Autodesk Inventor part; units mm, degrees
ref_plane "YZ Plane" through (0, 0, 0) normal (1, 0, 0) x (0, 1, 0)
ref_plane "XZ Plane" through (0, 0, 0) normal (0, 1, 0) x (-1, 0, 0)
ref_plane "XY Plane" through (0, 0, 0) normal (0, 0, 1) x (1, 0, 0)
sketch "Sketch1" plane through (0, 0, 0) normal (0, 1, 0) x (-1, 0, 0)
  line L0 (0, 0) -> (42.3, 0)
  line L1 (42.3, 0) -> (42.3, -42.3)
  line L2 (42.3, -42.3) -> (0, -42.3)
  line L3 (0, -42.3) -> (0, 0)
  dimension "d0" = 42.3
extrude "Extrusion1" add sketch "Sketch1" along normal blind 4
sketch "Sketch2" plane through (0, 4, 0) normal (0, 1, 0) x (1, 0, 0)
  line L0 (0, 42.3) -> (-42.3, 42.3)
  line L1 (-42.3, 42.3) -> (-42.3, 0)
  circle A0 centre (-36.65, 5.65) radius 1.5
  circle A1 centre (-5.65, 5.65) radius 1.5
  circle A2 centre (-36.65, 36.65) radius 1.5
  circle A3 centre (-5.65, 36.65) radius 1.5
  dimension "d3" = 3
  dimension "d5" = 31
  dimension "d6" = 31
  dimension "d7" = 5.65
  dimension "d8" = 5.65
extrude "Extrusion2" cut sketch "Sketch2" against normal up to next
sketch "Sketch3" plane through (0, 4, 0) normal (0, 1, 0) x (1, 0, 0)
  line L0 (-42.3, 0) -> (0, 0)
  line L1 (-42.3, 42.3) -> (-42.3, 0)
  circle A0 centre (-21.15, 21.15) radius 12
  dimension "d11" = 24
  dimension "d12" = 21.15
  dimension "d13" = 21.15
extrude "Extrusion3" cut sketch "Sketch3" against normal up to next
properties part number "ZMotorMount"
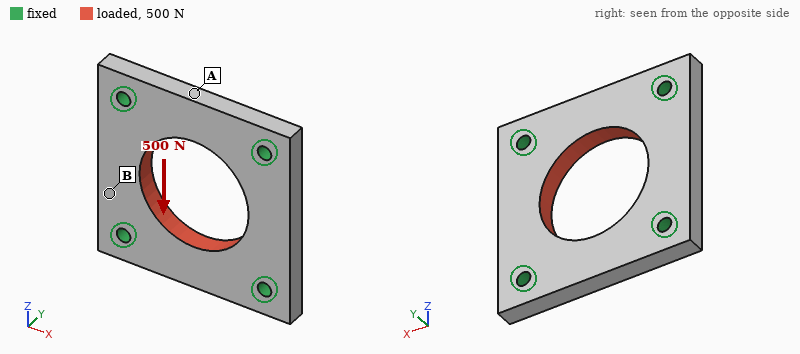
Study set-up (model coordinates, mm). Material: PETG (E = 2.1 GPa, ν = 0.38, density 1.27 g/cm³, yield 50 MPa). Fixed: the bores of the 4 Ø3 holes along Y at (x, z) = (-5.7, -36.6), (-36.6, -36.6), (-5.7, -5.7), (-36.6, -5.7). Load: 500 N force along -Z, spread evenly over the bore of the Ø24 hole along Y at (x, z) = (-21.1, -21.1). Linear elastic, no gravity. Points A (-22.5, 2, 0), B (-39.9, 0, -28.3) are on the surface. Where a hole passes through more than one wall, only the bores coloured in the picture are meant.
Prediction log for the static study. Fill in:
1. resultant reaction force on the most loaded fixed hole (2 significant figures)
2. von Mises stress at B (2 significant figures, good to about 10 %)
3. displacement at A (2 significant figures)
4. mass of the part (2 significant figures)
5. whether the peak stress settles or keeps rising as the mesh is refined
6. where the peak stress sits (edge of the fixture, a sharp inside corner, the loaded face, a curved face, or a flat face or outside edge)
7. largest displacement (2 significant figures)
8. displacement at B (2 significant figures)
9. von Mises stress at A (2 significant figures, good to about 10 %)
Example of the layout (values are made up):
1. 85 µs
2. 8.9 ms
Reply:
1. 130 N
2. 1.7 MPa
3. 37 µm
4. 6.6 g
5. keeps rising
6. edge of the fixture
7. 42 µm
8. 7.3 µm
9. 4.0 MPa
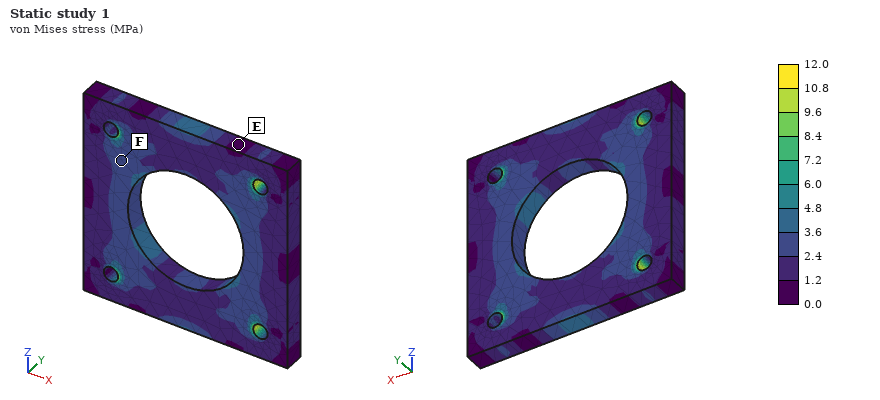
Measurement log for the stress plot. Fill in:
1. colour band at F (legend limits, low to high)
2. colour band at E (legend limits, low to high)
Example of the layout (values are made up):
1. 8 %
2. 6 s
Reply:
1. 2.4 to 3.6 MPa
2. 0.0 to 1.2 MPa
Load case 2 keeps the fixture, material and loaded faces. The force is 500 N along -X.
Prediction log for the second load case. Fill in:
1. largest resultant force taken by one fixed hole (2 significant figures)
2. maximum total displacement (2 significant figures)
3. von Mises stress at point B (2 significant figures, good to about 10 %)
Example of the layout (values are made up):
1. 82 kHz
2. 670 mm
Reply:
1. 130 N
2. 42 µm
3. 1.9 MPa
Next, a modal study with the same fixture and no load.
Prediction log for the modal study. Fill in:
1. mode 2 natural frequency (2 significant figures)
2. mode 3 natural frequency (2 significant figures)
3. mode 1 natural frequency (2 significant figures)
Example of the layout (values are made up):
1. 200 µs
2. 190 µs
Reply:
1. 5300 Hz
2. 5400 Hz
3. 5200 Hz
